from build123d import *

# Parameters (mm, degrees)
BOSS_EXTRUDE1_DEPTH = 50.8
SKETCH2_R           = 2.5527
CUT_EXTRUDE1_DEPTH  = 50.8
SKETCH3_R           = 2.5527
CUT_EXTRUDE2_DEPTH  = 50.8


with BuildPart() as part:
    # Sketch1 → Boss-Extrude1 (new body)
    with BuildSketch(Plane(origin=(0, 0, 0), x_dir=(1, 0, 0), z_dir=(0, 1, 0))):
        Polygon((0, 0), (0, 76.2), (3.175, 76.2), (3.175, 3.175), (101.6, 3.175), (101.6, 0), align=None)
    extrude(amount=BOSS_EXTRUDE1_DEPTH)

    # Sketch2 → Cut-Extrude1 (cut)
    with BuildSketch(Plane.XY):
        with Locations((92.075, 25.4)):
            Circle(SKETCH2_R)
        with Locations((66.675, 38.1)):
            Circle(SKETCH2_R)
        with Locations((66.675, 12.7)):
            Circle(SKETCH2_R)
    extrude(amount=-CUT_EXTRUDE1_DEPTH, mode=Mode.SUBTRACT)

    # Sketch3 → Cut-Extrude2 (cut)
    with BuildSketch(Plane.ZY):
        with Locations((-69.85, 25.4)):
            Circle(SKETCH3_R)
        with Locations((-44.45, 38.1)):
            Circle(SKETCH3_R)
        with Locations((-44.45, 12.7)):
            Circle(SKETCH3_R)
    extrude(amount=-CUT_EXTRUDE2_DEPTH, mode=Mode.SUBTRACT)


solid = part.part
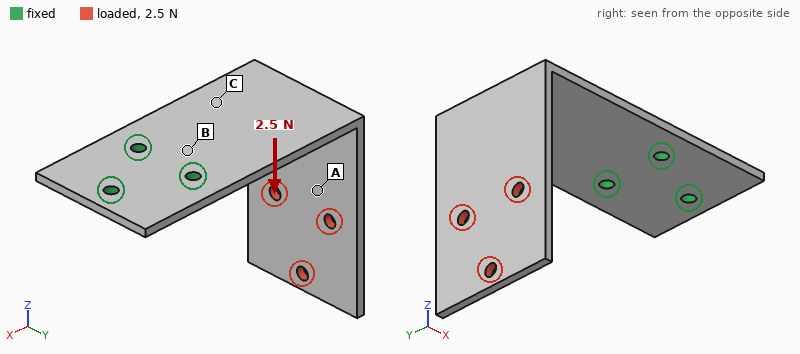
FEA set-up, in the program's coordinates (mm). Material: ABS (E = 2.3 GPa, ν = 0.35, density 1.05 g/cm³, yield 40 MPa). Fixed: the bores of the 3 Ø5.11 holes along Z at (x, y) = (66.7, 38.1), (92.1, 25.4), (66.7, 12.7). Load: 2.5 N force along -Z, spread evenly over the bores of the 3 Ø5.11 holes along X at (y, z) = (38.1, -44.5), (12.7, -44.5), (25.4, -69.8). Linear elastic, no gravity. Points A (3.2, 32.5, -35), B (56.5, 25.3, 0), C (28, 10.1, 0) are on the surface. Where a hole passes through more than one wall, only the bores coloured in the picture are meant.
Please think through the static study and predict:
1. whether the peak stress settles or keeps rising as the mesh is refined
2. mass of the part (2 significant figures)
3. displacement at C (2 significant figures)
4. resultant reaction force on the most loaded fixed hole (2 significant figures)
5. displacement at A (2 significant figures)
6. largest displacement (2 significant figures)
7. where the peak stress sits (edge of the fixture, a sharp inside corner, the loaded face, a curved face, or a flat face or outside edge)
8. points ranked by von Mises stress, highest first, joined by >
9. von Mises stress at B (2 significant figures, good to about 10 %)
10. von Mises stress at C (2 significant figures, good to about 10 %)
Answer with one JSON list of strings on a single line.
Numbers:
["keeps rising", "29 g", "0.29 mm", "1.6 N", "0.84 mm", "1.4 mm", "edge of the fixture", "B > C > A", "1.4 MPa", "0.75 MPa"]
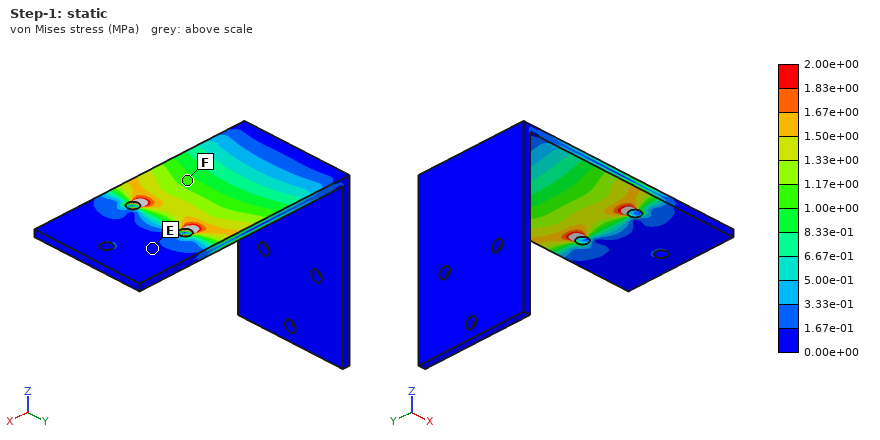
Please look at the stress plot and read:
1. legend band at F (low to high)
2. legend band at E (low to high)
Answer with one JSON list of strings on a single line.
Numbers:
["1.00e+00 to 1.17e+00 MPa", "0.00e+00 to 1.67e-01 MPa"]
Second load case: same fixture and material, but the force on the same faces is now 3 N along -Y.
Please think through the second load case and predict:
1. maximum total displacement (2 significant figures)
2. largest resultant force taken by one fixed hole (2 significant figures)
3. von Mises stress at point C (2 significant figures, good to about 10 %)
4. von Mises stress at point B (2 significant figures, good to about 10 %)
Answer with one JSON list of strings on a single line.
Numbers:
["1.3 mm", "7.7 N", "1.4 MPa", "0.85 MPa"]
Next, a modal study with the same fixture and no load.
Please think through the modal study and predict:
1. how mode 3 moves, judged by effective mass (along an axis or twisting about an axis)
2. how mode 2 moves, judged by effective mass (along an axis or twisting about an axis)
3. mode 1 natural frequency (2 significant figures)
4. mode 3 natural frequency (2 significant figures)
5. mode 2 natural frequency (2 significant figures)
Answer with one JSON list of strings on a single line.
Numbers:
["along Z", "along Y", "54 Hz", "150 Hz", "95 Hz"]
